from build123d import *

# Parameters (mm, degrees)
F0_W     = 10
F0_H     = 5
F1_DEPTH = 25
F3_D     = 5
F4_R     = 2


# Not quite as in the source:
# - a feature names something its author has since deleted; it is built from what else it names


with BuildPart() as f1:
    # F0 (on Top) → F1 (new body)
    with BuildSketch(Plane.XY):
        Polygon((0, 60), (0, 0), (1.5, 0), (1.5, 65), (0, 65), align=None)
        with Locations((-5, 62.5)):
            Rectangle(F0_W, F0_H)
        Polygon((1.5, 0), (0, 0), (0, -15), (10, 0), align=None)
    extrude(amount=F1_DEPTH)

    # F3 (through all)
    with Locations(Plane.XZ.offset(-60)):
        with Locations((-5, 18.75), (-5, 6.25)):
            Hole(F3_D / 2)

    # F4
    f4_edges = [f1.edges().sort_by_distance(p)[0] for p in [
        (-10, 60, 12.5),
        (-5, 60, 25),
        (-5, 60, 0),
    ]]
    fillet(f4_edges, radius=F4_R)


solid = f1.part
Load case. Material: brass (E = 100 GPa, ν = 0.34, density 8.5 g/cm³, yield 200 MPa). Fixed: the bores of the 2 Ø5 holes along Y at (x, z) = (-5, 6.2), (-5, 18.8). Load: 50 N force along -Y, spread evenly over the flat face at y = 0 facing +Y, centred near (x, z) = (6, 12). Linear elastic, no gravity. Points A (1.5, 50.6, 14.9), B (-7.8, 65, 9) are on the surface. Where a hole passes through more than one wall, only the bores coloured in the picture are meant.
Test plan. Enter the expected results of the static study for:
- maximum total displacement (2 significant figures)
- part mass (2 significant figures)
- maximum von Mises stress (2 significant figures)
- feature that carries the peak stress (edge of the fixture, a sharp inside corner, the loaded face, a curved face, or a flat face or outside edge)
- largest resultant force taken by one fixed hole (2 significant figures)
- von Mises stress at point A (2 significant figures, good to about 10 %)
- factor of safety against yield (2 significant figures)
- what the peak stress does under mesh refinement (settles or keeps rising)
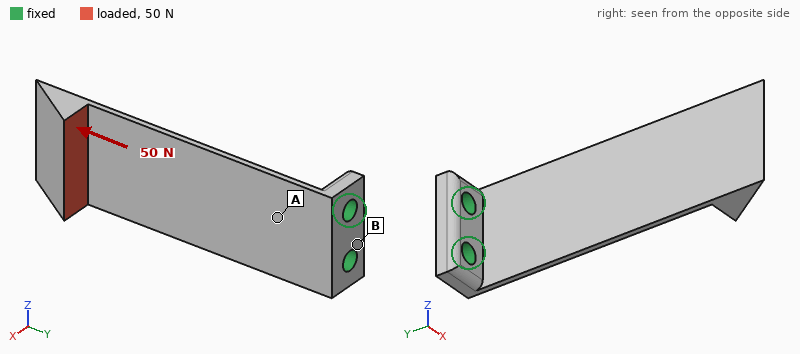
0.96 mm
45 g
29 MPa
a flat face or outside edge
25 N
26 MPa
6.9
settles
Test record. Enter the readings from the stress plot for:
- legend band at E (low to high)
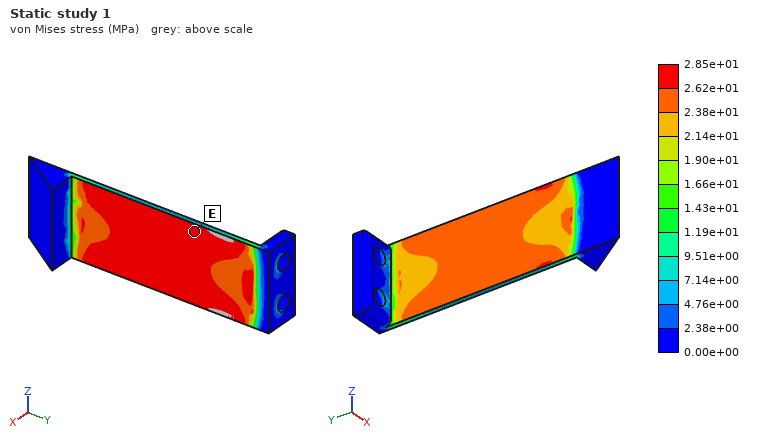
2.62e+01 to 2.85e+01 MPa
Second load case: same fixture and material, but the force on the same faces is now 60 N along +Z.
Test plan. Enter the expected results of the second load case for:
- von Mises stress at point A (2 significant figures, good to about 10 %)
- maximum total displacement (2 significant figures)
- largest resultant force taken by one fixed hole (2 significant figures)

27 MPa
0.25 mm
220 N
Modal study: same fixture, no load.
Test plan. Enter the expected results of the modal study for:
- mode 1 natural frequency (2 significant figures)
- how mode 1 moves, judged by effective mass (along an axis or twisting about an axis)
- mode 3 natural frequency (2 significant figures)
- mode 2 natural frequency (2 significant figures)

100 Hz
along X
840 Hz
610 Hz
